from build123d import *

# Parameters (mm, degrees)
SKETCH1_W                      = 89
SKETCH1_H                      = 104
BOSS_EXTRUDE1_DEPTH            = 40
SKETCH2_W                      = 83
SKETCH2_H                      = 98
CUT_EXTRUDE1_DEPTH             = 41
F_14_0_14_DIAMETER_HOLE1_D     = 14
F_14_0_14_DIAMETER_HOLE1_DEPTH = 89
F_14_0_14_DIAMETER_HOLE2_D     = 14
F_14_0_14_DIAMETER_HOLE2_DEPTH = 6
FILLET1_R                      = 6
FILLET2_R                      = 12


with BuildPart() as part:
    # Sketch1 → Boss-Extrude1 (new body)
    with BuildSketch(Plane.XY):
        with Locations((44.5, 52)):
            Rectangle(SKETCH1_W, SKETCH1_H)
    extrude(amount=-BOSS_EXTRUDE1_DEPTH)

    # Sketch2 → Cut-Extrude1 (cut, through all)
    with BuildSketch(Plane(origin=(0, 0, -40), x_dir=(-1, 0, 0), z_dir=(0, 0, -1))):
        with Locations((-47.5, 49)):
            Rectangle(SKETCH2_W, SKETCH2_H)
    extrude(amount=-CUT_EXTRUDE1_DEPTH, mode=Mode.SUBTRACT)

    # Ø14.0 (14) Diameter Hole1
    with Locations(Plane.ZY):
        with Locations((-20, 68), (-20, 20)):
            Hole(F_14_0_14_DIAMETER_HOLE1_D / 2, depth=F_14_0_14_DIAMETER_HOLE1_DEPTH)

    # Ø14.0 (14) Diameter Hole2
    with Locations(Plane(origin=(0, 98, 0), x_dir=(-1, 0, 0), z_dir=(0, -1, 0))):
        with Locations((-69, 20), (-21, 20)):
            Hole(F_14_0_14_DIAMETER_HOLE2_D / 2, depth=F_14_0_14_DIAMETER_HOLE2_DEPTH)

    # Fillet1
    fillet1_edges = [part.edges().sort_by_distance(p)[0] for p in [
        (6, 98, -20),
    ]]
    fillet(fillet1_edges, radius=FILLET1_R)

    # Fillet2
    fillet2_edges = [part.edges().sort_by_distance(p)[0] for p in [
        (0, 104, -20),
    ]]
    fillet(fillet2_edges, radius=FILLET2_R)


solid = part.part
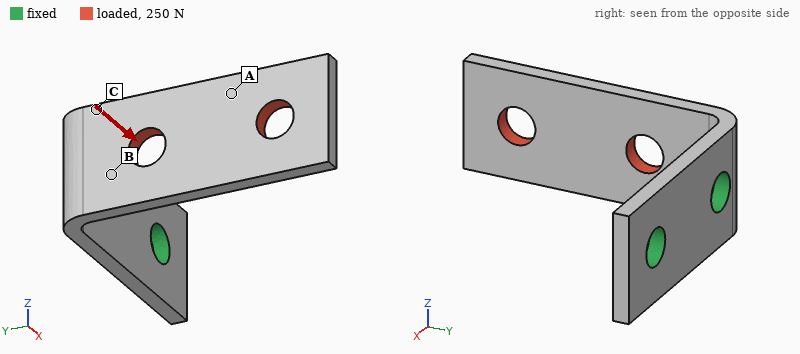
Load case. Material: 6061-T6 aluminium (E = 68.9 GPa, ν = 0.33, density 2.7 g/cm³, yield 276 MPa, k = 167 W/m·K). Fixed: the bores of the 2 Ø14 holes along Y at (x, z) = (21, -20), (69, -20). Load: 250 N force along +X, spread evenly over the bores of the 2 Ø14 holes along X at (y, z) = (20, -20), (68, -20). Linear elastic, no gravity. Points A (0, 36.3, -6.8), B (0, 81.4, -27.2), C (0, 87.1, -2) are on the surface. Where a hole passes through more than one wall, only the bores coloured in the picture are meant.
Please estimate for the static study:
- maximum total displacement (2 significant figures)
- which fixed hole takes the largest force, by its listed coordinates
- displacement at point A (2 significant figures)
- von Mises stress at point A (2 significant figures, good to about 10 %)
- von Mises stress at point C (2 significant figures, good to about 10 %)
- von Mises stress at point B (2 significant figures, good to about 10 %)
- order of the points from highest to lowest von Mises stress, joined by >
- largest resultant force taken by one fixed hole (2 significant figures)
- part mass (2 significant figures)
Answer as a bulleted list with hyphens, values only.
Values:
- 1.1 mm
- (21, -20)
- 0.59 mm
- 9.2 MPa
- 48 MPa
- 35 MPa
- C > B > A
- 250 N
- 110 g
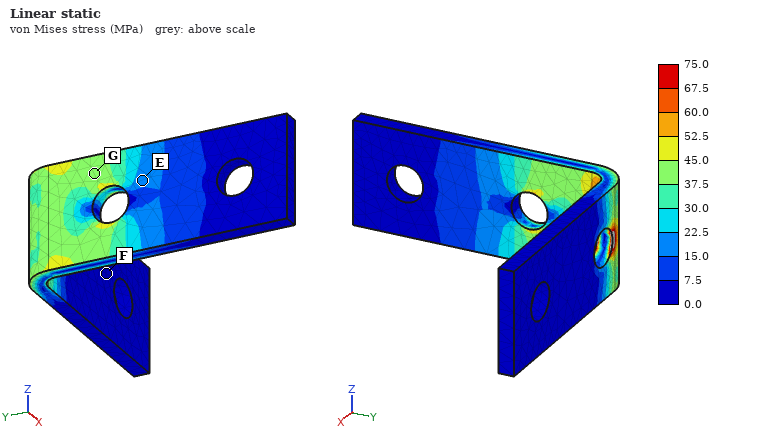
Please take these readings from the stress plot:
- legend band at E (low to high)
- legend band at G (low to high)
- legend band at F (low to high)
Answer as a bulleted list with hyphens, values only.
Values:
- 15.0 to 22.5 MPa
- 37.5 to 45.0 MPa
- 0.0 to 7.5 MPa
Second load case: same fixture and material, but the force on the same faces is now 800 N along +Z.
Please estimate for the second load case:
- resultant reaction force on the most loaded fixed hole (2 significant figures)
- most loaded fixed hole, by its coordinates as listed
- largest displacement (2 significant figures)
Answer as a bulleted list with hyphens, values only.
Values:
- 890 N
- (21, -20)
- 0.59 mm
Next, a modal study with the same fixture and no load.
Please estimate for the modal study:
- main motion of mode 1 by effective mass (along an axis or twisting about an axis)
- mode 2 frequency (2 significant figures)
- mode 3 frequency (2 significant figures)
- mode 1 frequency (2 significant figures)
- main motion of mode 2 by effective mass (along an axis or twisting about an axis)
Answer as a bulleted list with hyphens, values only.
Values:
- along X
- 980 Hz
- 2200 Hz
- 420 Hz
- along Z
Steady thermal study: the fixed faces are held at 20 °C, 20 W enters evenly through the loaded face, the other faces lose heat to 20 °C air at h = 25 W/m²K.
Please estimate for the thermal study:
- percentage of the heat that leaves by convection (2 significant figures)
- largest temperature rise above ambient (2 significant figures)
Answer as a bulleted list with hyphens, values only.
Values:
- 23 %
- 30 K
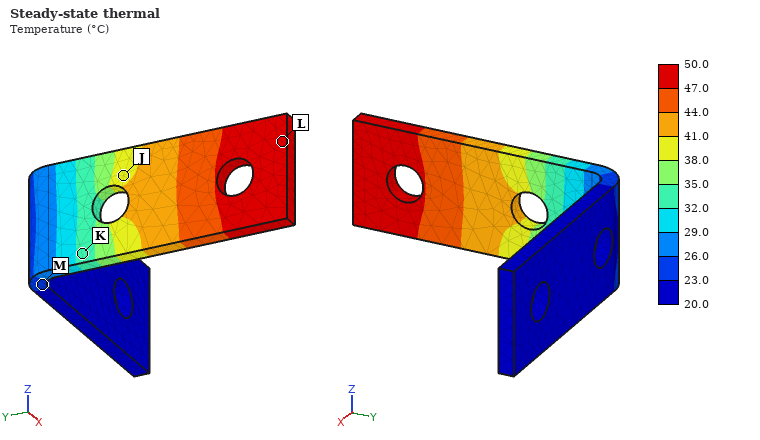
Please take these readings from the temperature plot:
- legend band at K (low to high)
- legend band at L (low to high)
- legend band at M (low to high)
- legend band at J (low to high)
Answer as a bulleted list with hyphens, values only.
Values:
- 32.0 to 35.0 °C
- 47.0 to 50.0 °C
- 23.0 to 26.0 °C
- 38.0 to 41.0 °C
